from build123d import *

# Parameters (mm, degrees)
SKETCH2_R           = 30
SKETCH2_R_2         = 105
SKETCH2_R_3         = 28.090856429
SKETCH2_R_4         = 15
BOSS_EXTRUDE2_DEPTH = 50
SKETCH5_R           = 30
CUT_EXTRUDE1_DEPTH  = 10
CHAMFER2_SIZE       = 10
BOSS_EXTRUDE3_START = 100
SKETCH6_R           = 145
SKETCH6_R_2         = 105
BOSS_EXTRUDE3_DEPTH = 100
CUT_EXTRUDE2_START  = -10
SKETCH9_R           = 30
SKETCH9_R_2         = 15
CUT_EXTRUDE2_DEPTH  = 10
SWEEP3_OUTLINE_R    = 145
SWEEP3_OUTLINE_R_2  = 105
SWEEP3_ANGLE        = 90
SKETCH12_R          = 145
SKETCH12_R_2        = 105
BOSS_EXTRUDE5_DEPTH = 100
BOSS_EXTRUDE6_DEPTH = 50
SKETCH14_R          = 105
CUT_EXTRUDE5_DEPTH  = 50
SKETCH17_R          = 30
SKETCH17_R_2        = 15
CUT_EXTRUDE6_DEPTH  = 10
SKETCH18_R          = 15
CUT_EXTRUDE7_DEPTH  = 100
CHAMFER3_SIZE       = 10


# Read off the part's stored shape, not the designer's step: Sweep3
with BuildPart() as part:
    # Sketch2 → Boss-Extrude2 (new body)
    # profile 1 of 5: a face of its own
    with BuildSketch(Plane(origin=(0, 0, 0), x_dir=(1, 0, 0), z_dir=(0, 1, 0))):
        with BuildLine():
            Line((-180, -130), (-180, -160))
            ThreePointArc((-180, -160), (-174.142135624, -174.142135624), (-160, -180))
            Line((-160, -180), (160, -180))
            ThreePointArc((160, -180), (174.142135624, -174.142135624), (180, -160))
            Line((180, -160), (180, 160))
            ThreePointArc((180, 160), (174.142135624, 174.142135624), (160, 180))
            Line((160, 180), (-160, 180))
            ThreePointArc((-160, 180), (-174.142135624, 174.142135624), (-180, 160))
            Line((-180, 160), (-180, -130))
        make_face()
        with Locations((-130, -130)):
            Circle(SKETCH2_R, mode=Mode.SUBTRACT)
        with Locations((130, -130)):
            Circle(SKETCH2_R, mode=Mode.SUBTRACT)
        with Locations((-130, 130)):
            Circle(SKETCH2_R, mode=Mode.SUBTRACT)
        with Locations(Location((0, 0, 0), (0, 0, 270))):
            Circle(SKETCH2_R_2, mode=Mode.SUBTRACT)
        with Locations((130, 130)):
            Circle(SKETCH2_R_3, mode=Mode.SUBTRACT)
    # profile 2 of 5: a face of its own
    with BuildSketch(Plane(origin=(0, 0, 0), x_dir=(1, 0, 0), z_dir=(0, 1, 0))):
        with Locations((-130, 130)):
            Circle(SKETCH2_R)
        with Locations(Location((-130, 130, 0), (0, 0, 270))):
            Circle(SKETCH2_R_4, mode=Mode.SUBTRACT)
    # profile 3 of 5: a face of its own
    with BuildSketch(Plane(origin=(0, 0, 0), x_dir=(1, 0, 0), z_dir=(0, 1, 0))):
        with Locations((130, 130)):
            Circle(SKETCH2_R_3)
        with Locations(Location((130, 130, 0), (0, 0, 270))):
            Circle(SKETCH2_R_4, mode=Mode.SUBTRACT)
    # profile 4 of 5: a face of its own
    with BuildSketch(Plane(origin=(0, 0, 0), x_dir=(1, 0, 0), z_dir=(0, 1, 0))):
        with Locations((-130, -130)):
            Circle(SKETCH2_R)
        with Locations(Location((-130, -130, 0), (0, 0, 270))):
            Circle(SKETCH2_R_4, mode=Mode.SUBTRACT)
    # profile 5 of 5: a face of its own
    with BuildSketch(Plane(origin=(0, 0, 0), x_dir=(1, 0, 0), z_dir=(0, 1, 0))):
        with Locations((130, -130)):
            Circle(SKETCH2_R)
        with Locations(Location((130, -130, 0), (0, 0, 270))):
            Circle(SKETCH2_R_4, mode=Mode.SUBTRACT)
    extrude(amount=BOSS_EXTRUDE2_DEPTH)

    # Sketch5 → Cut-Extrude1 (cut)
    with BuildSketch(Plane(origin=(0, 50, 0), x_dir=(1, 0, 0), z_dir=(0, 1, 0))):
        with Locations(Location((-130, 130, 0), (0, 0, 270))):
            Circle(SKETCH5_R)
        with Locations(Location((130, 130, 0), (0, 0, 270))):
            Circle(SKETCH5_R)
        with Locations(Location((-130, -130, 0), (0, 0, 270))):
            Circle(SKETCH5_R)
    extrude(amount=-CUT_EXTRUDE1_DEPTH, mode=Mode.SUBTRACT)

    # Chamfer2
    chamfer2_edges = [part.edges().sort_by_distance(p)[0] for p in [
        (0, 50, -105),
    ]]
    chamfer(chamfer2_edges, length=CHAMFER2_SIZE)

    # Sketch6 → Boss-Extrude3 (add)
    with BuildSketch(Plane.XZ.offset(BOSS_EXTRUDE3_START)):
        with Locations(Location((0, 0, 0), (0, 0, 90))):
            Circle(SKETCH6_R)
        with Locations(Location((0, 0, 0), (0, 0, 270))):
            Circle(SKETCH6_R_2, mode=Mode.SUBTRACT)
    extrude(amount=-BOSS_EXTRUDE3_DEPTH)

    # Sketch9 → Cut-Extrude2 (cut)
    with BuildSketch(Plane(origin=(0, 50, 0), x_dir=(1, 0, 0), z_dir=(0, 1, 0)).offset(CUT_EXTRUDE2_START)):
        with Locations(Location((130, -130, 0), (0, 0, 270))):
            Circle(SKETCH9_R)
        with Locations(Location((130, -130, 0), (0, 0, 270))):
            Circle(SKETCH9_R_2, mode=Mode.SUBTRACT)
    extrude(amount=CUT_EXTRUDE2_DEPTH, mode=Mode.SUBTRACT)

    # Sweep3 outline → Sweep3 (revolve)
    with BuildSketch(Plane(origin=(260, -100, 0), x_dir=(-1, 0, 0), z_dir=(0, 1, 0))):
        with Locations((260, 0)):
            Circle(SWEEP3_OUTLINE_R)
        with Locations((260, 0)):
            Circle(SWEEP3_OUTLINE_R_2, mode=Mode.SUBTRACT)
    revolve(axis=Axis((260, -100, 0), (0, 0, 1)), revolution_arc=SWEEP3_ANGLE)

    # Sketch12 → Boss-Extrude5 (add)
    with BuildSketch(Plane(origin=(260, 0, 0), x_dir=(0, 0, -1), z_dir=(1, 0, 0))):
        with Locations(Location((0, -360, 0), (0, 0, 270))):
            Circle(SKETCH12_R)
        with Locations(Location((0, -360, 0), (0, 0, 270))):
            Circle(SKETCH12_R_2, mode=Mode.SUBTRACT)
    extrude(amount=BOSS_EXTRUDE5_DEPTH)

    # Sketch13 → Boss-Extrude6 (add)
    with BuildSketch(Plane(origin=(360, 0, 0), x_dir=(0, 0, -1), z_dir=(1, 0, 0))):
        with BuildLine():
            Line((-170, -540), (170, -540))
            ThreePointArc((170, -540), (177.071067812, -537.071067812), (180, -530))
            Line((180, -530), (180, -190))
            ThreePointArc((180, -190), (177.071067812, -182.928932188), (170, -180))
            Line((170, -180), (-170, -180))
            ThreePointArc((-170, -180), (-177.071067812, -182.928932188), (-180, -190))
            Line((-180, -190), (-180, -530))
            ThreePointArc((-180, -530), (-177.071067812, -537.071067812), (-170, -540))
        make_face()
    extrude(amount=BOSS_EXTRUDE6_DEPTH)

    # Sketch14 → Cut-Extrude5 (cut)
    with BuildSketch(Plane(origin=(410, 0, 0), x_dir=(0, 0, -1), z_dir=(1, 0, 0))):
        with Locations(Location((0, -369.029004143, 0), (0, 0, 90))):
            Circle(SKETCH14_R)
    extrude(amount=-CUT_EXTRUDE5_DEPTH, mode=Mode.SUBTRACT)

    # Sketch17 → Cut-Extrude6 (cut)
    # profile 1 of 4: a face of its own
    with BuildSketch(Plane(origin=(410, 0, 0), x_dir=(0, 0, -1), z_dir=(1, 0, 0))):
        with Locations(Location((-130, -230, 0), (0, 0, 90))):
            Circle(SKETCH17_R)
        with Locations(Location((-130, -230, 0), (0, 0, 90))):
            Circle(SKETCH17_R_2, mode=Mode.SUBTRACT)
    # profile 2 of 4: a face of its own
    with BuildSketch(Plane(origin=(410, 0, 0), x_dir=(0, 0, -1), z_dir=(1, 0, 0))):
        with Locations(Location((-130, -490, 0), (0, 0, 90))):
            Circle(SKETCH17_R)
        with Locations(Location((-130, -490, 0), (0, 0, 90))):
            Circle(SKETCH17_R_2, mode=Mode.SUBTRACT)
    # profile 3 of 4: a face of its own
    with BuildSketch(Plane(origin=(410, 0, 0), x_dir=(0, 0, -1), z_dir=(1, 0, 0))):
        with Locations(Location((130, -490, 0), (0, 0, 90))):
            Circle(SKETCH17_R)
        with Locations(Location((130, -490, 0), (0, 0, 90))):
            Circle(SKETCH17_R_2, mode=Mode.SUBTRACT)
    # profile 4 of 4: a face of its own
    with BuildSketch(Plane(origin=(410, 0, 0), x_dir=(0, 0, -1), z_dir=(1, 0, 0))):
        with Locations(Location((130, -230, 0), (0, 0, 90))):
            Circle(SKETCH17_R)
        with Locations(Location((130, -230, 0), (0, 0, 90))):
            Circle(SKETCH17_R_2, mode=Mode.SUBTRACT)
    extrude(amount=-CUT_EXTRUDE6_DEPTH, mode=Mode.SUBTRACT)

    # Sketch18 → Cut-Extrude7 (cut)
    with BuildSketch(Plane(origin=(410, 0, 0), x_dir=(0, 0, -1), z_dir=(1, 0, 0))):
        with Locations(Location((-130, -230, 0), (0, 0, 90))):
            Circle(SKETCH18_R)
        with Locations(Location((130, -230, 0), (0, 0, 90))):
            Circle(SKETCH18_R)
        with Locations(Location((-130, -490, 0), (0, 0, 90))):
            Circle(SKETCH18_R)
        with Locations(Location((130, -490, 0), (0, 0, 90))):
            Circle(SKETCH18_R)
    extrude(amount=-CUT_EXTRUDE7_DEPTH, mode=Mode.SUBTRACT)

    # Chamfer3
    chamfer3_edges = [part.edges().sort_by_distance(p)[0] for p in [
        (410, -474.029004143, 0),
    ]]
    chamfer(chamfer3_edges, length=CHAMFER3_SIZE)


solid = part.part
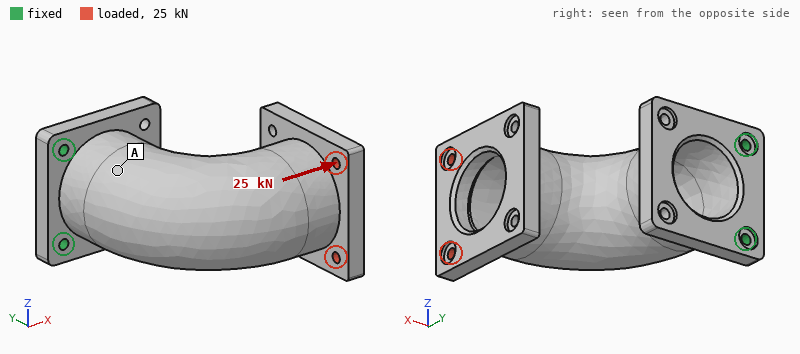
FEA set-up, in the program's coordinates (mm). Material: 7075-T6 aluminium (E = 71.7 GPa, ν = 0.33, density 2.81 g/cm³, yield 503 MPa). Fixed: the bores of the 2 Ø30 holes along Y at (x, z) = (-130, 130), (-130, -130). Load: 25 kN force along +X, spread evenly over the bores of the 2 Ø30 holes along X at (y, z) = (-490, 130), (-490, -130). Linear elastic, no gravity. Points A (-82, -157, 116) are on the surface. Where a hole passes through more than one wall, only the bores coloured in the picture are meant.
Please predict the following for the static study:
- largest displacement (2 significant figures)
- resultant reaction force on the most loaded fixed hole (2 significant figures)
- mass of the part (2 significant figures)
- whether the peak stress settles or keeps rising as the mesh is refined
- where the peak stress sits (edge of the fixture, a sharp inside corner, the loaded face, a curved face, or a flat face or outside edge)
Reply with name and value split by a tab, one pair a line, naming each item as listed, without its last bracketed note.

largest displacement	3.9 mm
resultant reaction force on the most loaded fixed hole	13 kN
mass of the part	79 kg
whether the peak stress settles or keeps rising as the mesh is refined	keeps rising
where the peak stress sits	edge of the fixture
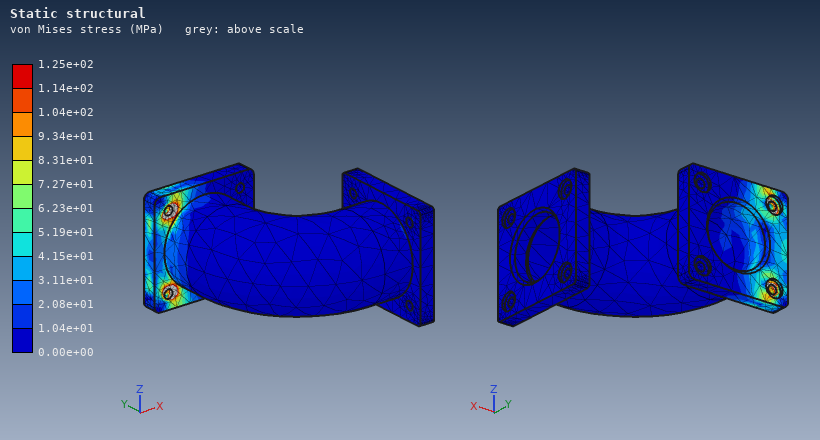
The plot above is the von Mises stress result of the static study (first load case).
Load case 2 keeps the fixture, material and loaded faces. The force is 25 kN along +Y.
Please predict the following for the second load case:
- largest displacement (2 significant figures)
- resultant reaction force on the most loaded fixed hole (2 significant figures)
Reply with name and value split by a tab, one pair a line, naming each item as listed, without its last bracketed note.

largest displacement	3.7 mm
resultant reaction force on the most loaded fixed hole	13 kN
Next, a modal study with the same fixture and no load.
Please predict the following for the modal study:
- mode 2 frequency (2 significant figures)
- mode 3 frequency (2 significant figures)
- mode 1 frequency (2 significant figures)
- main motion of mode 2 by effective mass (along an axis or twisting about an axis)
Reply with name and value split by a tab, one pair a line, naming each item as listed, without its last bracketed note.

mode 2 frequency	220 Hz
mode 3 frequency	540 Hz
mode 1 frequency	68 Hz
main motion of mode 2 by effective mass	along Z
